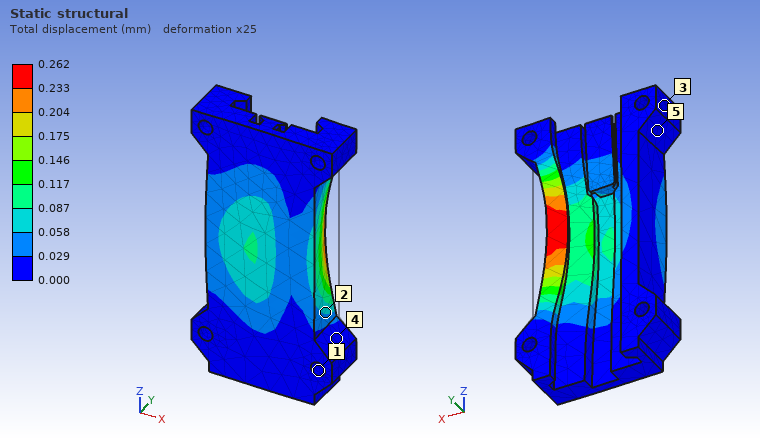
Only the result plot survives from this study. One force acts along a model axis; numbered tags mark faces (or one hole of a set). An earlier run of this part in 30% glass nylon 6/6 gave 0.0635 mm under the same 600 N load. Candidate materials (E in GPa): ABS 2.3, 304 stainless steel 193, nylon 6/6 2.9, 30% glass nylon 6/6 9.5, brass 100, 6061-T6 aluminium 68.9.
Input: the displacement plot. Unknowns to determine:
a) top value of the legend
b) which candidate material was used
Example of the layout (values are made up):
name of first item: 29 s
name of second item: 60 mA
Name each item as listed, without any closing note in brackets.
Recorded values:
top value of the legend: 0.262 mm
which candidate material was used: ABS
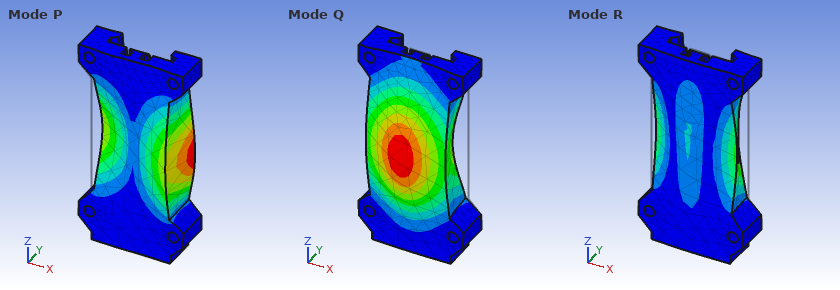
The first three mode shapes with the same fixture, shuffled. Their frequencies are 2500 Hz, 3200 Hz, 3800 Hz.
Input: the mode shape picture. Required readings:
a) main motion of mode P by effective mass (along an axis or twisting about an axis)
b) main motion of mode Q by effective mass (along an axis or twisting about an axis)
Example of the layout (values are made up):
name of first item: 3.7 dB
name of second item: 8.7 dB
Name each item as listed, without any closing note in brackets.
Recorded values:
main motion of mode P by effective mass: along X
main motion of mode Q by effective mass: along Y
